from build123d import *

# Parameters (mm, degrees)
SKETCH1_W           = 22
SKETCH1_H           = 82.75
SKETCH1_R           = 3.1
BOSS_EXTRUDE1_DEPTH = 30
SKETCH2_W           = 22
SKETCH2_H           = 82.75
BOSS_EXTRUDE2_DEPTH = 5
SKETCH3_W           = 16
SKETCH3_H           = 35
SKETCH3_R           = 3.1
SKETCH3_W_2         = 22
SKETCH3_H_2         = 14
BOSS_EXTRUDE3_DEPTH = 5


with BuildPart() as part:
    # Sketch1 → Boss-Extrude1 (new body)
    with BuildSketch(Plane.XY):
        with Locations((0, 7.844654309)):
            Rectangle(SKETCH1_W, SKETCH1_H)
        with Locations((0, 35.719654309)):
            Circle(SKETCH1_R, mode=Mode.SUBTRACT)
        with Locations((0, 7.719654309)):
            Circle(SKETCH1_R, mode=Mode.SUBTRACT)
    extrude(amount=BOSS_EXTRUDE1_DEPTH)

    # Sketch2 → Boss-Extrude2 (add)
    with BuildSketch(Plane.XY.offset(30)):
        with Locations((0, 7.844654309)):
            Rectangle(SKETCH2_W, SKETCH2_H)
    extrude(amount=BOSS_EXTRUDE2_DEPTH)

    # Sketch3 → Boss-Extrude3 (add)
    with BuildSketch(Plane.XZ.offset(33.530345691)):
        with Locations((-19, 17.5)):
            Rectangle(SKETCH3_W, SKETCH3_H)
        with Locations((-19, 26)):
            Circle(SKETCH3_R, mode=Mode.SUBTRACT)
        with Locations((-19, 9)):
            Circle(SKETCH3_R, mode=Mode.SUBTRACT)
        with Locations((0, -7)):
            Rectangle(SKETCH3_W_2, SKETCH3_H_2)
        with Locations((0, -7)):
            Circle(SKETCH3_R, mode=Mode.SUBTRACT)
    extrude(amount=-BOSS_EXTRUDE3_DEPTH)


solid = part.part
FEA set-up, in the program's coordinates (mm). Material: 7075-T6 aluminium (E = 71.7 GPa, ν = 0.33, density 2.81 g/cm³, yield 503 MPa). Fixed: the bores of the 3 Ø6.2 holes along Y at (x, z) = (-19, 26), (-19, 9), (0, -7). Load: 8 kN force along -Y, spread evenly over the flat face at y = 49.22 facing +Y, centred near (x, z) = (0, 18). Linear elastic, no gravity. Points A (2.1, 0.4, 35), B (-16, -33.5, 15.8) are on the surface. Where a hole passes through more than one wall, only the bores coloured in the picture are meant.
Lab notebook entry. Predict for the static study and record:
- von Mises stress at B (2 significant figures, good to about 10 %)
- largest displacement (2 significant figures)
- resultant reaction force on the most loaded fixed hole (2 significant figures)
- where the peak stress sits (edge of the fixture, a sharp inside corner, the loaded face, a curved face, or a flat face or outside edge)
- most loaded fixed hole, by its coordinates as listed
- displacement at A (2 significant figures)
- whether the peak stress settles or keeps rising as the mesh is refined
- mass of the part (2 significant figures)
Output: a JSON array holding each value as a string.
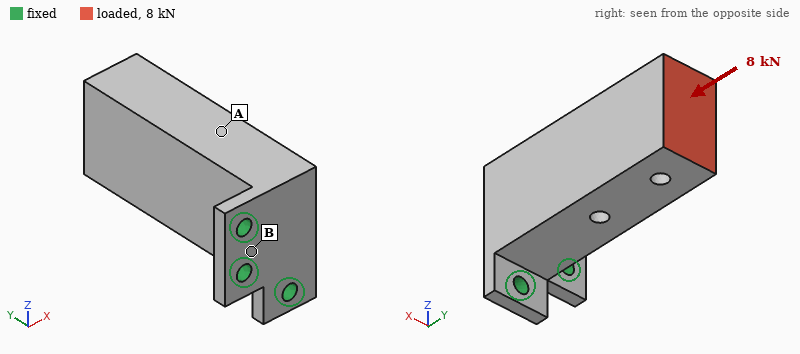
["110 MPa", "0.69 mm", "5.4 kN", "edge of the fixture", "(-19, 26)", "0.32 mm", "keeps rising", "180 g"]
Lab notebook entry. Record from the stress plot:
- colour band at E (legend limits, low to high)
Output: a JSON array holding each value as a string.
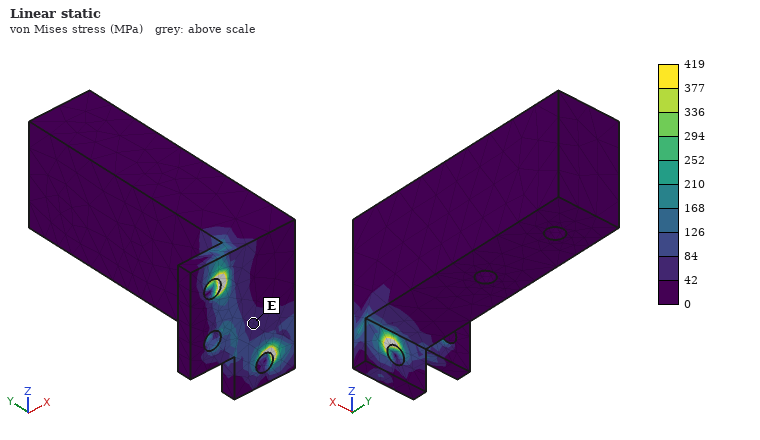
["42 to 84 MPa"]
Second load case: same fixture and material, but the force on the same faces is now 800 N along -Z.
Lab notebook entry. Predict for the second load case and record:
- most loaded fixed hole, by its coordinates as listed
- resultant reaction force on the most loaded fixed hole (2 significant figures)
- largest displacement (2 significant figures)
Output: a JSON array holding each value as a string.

["(-19, 26)", "2.4 kN", "0.26 mm"]
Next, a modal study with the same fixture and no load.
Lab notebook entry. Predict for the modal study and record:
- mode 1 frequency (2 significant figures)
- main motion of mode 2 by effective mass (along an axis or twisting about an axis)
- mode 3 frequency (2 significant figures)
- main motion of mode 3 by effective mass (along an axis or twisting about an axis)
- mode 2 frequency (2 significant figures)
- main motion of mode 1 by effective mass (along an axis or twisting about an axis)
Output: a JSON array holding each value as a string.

["820 Hz", "along Z", "6300 Hz", "along Y", "1900 Hz", "along X"]
